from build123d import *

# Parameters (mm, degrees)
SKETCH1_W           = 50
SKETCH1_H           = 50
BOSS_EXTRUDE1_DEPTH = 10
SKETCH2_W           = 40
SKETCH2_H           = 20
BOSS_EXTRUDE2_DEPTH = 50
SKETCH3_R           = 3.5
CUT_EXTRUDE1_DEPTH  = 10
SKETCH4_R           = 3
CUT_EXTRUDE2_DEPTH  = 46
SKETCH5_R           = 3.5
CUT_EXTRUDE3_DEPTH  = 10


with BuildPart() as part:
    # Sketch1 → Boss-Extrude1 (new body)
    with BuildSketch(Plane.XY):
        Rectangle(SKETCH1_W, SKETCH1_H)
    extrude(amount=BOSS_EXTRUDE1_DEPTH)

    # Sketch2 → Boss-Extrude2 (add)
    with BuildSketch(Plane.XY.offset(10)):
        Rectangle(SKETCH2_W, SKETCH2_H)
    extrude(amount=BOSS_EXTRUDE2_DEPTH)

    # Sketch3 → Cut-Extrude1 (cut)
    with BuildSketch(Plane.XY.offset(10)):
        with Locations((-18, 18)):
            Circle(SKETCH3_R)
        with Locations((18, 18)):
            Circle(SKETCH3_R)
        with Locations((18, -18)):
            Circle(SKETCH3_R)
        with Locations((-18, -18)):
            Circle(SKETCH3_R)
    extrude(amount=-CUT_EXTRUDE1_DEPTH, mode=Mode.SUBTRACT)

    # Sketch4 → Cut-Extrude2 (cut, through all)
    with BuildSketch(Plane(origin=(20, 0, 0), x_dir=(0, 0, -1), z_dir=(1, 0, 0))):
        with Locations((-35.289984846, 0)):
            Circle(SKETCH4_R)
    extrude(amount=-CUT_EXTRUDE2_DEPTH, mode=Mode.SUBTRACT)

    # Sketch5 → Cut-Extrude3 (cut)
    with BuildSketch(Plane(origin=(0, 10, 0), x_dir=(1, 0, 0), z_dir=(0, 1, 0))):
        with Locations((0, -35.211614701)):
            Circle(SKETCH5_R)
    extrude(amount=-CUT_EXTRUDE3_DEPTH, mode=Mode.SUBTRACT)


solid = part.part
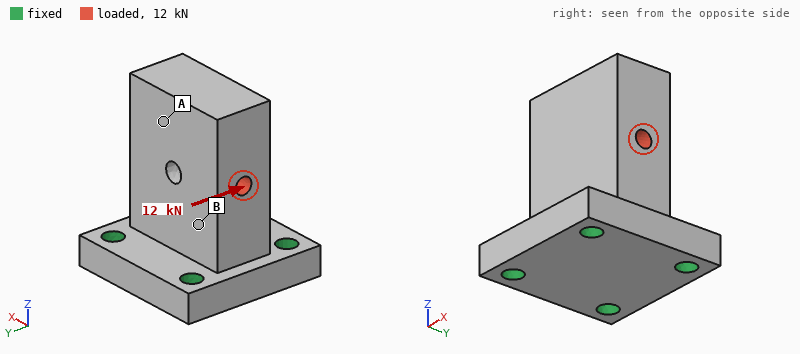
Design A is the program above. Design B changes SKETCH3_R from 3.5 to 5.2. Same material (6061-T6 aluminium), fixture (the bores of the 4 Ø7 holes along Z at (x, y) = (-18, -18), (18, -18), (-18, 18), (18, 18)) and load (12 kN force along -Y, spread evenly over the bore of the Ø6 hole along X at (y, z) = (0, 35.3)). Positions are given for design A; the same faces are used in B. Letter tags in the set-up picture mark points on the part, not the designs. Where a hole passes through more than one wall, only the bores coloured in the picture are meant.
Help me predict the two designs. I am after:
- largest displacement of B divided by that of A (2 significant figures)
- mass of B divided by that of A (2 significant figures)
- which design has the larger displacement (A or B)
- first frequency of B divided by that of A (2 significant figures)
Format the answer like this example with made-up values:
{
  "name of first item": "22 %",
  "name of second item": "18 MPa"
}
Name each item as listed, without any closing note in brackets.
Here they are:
{
  "largest displacement of B divided by that of A": "0.91",
  "mass of B divided by that of A": "0.97",
  "which design has the larger displacement": "A",
  "first frequency of B divided by that of A": "1.0"
}
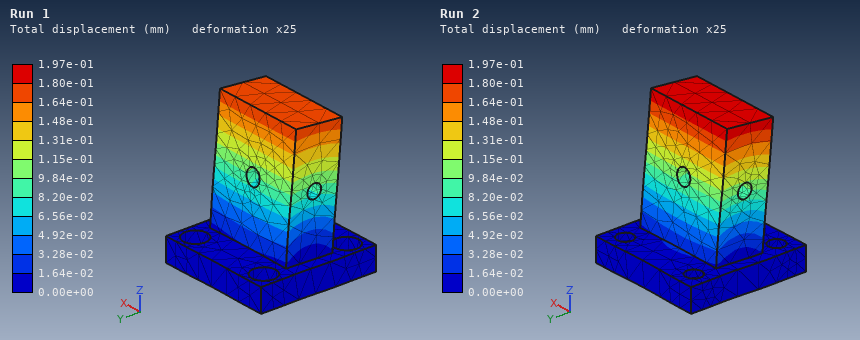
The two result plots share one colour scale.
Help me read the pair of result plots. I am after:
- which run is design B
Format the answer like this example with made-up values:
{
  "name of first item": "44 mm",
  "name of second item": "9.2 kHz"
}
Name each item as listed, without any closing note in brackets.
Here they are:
{
  "which run is design B": "Run 1"
}
